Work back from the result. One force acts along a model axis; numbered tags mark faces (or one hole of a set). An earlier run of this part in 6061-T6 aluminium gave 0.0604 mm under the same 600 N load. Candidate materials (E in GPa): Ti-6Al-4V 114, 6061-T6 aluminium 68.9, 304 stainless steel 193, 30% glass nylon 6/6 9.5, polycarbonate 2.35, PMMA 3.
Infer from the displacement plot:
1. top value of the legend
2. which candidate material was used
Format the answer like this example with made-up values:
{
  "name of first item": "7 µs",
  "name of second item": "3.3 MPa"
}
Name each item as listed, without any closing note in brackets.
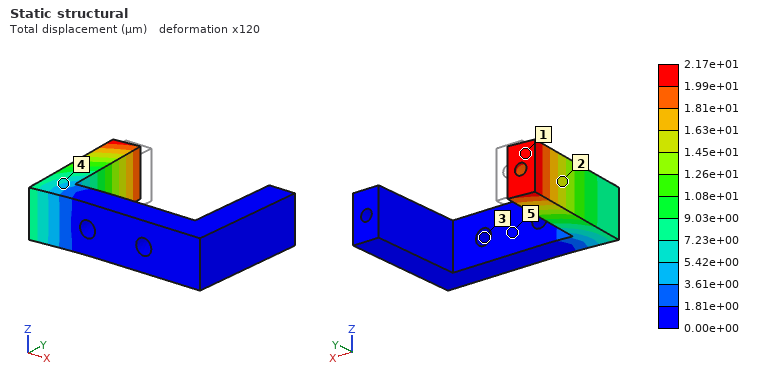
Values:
{
  "top value of the legend": "2.17e+01 µm",
  "which candidate material was used": "304 stainless steel"
}
